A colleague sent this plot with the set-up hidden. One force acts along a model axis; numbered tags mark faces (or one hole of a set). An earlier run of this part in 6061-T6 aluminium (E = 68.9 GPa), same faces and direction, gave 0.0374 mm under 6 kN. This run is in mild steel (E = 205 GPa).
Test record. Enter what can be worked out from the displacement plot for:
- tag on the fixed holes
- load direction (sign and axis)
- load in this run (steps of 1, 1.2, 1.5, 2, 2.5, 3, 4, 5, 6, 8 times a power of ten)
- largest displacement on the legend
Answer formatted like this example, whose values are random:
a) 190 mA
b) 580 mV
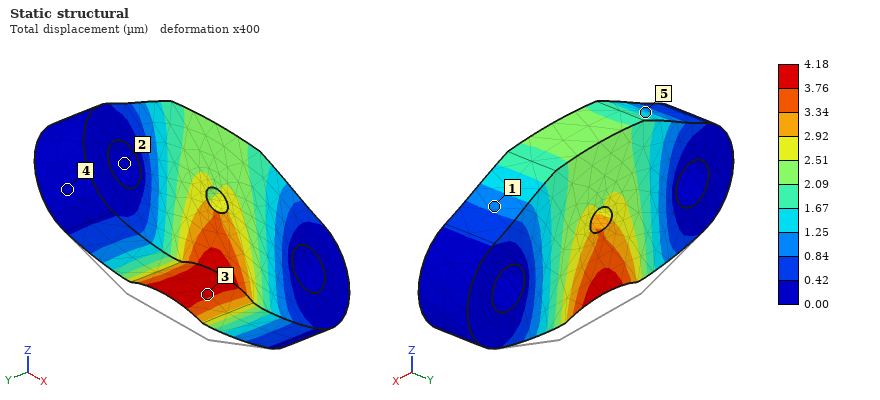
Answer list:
a) 2
b) +Z
c) 2 kN
d) 4.18 µm
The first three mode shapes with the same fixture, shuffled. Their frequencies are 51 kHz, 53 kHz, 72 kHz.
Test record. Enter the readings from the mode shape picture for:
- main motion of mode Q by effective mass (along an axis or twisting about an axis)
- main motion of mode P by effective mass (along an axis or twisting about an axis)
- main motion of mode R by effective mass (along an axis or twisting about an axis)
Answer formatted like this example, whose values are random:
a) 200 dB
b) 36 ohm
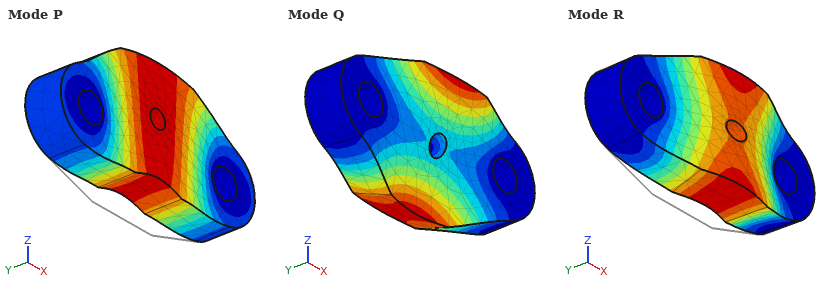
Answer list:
a) twisting about X
b) along Z
c) along Y
